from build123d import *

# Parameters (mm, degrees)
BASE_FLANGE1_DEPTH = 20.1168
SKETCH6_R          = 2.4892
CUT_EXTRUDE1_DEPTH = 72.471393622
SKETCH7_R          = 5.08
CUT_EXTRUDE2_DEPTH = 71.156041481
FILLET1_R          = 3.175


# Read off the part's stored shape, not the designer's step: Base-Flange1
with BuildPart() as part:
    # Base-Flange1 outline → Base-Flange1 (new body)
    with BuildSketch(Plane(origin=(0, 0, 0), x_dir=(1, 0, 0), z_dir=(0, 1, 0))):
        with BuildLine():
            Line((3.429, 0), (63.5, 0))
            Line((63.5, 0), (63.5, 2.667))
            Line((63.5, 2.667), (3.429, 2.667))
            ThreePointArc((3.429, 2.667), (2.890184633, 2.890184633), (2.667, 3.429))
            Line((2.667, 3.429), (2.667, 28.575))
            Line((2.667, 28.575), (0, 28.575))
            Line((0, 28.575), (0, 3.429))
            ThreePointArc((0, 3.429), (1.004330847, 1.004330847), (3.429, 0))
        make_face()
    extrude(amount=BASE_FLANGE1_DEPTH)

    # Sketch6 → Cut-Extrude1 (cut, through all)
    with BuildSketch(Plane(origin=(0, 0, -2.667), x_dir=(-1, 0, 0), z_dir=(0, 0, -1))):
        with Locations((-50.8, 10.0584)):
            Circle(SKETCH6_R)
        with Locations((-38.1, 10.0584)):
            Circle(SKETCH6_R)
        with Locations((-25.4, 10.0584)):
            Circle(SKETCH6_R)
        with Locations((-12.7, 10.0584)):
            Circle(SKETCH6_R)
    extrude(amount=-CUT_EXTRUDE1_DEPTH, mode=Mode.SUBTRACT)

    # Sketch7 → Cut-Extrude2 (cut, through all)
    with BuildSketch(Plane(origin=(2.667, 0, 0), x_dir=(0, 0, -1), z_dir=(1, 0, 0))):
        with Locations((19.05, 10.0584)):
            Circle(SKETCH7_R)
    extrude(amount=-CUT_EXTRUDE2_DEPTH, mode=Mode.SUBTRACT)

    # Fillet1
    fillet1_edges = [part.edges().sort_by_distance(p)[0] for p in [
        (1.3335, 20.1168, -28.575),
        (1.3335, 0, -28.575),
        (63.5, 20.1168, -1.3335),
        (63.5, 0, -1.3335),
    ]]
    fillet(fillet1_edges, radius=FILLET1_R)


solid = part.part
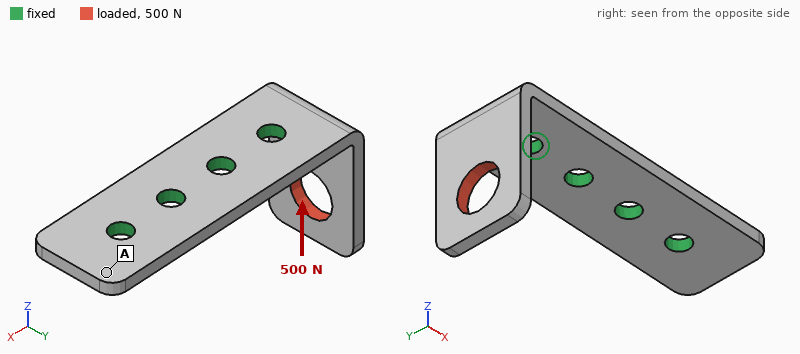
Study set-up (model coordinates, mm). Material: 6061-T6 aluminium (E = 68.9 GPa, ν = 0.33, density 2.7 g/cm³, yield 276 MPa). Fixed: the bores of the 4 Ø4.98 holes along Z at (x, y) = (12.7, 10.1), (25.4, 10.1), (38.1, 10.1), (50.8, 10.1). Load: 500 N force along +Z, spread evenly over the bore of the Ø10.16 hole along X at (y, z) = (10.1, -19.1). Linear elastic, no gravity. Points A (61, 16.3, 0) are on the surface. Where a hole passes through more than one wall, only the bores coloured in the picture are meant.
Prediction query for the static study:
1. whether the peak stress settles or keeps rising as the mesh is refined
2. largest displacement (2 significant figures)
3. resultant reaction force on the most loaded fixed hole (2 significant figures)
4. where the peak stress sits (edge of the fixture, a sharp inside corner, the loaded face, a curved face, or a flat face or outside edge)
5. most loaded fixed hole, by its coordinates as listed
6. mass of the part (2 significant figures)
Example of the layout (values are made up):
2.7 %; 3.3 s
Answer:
keeps rising; 0.34 mm; 580 N; edge of the fixture; (12.7, 10.1); 12 g
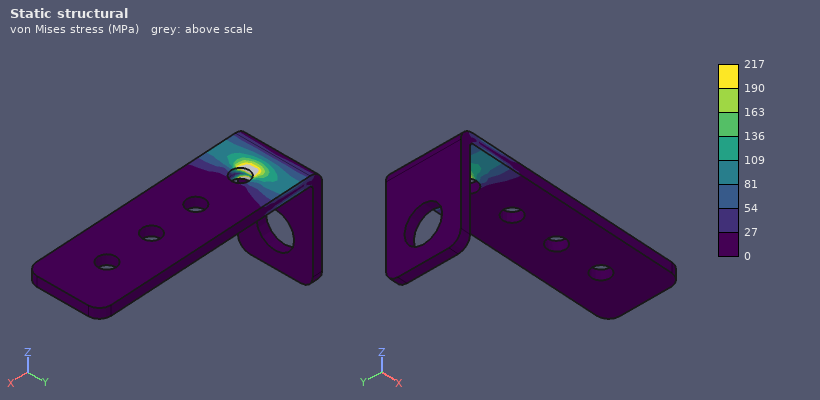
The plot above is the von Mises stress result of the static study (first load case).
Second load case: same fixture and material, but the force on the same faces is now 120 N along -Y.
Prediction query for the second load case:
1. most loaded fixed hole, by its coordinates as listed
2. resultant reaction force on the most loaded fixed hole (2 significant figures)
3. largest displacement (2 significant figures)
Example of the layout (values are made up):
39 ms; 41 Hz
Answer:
(12.7, 10.1); 170 N; 0.15 mm
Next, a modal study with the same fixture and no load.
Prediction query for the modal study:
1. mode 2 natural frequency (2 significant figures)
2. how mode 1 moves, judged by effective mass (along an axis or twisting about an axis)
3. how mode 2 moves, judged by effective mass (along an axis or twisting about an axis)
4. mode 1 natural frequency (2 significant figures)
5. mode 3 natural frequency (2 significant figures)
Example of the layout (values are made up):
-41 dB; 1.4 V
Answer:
3300 Hz; along X; along Y; 2100 Hz; 7700 Hz
